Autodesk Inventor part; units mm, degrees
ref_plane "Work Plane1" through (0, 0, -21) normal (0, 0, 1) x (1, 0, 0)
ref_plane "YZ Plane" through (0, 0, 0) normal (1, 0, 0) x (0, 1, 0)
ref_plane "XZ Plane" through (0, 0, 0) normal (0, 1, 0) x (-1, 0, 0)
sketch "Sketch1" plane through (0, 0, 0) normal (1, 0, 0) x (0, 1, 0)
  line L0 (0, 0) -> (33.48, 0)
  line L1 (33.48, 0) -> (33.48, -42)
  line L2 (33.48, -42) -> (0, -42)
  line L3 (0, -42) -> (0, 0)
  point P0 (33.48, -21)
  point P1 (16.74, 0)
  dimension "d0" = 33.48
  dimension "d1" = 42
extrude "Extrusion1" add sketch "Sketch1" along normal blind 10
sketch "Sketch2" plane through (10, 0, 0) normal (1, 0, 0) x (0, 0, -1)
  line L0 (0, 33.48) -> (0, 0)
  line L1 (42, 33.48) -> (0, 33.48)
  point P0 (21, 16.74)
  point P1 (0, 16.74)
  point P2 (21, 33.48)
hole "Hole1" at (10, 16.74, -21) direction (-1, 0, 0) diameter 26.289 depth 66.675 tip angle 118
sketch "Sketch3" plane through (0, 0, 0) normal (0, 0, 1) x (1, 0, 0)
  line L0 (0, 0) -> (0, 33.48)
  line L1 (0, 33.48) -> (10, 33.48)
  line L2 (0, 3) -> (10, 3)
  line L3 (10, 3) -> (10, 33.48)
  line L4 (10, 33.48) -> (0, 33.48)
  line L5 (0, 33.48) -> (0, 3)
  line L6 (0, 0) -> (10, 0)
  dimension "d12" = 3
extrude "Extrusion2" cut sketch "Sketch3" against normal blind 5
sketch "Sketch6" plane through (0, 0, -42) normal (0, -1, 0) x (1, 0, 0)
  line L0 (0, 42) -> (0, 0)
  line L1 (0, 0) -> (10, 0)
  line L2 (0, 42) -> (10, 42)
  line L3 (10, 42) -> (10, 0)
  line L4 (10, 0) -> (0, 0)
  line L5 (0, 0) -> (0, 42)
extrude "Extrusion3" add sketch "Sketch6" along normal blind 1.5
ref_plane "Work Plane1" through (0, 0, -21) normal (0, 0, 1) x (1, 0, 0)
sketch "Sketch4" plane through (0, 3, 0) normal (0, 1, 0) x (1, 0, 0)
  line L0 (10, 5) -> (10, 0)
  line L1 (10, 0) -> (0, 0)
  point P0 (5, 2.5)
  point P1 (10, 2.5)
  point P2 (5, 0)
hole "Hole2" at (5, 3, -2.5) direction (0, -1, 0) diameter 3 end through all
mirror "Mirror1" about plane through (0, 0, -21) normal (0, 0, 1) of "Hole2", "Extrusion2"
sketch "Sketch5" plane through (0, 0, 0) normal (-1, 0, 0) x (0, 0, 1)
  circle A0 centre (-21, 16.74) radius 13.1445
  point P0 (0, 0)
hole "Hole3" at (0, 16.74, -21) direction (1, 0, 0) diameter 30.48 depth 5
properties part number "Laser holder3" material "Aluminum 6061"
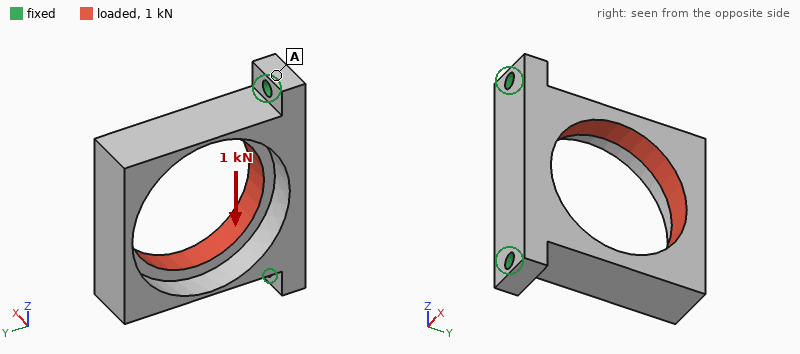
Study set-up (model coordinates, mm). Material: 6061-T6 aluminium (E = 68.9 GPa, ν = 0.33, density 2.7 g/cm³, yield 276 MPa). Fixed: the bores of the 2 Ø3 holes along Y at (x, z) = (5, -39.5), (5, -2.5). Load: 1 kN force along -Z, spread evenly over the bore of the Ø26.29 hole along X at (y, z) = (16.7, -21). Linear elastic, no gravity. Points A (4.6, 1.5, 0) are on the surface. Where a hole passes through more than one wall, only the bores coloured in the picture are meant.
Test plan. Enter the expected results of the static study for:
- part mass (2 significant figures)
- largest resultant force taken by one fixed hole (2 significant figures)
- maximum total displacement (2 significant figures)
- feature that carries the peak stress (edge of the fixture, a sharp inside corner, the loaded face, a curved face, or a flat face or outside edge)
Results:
14 g
670 N
0.11 mm
the loaded face
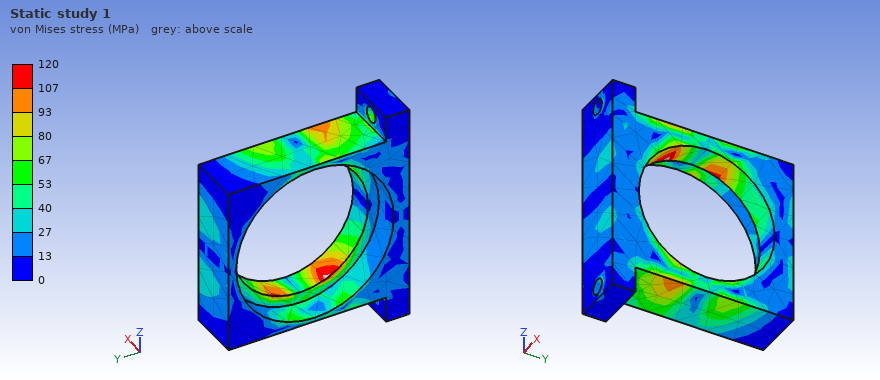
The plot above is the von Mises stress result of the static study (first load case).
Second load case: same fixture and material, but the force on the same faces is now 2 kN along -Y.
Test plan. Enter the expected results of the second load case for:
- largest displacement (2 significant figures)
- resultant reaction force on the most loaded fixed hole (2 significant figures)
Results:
87 µm
1.0 kN
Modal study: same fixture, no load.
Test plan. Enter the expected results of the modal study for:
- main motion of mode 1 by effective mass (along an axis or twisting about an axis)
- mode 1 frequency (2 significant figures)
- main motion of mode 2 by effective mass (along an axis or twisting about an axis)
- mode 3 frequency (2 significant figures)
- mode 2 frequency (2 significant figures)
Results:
along X
3000 Hz
along Z
6400 Hz
4500 Hz
